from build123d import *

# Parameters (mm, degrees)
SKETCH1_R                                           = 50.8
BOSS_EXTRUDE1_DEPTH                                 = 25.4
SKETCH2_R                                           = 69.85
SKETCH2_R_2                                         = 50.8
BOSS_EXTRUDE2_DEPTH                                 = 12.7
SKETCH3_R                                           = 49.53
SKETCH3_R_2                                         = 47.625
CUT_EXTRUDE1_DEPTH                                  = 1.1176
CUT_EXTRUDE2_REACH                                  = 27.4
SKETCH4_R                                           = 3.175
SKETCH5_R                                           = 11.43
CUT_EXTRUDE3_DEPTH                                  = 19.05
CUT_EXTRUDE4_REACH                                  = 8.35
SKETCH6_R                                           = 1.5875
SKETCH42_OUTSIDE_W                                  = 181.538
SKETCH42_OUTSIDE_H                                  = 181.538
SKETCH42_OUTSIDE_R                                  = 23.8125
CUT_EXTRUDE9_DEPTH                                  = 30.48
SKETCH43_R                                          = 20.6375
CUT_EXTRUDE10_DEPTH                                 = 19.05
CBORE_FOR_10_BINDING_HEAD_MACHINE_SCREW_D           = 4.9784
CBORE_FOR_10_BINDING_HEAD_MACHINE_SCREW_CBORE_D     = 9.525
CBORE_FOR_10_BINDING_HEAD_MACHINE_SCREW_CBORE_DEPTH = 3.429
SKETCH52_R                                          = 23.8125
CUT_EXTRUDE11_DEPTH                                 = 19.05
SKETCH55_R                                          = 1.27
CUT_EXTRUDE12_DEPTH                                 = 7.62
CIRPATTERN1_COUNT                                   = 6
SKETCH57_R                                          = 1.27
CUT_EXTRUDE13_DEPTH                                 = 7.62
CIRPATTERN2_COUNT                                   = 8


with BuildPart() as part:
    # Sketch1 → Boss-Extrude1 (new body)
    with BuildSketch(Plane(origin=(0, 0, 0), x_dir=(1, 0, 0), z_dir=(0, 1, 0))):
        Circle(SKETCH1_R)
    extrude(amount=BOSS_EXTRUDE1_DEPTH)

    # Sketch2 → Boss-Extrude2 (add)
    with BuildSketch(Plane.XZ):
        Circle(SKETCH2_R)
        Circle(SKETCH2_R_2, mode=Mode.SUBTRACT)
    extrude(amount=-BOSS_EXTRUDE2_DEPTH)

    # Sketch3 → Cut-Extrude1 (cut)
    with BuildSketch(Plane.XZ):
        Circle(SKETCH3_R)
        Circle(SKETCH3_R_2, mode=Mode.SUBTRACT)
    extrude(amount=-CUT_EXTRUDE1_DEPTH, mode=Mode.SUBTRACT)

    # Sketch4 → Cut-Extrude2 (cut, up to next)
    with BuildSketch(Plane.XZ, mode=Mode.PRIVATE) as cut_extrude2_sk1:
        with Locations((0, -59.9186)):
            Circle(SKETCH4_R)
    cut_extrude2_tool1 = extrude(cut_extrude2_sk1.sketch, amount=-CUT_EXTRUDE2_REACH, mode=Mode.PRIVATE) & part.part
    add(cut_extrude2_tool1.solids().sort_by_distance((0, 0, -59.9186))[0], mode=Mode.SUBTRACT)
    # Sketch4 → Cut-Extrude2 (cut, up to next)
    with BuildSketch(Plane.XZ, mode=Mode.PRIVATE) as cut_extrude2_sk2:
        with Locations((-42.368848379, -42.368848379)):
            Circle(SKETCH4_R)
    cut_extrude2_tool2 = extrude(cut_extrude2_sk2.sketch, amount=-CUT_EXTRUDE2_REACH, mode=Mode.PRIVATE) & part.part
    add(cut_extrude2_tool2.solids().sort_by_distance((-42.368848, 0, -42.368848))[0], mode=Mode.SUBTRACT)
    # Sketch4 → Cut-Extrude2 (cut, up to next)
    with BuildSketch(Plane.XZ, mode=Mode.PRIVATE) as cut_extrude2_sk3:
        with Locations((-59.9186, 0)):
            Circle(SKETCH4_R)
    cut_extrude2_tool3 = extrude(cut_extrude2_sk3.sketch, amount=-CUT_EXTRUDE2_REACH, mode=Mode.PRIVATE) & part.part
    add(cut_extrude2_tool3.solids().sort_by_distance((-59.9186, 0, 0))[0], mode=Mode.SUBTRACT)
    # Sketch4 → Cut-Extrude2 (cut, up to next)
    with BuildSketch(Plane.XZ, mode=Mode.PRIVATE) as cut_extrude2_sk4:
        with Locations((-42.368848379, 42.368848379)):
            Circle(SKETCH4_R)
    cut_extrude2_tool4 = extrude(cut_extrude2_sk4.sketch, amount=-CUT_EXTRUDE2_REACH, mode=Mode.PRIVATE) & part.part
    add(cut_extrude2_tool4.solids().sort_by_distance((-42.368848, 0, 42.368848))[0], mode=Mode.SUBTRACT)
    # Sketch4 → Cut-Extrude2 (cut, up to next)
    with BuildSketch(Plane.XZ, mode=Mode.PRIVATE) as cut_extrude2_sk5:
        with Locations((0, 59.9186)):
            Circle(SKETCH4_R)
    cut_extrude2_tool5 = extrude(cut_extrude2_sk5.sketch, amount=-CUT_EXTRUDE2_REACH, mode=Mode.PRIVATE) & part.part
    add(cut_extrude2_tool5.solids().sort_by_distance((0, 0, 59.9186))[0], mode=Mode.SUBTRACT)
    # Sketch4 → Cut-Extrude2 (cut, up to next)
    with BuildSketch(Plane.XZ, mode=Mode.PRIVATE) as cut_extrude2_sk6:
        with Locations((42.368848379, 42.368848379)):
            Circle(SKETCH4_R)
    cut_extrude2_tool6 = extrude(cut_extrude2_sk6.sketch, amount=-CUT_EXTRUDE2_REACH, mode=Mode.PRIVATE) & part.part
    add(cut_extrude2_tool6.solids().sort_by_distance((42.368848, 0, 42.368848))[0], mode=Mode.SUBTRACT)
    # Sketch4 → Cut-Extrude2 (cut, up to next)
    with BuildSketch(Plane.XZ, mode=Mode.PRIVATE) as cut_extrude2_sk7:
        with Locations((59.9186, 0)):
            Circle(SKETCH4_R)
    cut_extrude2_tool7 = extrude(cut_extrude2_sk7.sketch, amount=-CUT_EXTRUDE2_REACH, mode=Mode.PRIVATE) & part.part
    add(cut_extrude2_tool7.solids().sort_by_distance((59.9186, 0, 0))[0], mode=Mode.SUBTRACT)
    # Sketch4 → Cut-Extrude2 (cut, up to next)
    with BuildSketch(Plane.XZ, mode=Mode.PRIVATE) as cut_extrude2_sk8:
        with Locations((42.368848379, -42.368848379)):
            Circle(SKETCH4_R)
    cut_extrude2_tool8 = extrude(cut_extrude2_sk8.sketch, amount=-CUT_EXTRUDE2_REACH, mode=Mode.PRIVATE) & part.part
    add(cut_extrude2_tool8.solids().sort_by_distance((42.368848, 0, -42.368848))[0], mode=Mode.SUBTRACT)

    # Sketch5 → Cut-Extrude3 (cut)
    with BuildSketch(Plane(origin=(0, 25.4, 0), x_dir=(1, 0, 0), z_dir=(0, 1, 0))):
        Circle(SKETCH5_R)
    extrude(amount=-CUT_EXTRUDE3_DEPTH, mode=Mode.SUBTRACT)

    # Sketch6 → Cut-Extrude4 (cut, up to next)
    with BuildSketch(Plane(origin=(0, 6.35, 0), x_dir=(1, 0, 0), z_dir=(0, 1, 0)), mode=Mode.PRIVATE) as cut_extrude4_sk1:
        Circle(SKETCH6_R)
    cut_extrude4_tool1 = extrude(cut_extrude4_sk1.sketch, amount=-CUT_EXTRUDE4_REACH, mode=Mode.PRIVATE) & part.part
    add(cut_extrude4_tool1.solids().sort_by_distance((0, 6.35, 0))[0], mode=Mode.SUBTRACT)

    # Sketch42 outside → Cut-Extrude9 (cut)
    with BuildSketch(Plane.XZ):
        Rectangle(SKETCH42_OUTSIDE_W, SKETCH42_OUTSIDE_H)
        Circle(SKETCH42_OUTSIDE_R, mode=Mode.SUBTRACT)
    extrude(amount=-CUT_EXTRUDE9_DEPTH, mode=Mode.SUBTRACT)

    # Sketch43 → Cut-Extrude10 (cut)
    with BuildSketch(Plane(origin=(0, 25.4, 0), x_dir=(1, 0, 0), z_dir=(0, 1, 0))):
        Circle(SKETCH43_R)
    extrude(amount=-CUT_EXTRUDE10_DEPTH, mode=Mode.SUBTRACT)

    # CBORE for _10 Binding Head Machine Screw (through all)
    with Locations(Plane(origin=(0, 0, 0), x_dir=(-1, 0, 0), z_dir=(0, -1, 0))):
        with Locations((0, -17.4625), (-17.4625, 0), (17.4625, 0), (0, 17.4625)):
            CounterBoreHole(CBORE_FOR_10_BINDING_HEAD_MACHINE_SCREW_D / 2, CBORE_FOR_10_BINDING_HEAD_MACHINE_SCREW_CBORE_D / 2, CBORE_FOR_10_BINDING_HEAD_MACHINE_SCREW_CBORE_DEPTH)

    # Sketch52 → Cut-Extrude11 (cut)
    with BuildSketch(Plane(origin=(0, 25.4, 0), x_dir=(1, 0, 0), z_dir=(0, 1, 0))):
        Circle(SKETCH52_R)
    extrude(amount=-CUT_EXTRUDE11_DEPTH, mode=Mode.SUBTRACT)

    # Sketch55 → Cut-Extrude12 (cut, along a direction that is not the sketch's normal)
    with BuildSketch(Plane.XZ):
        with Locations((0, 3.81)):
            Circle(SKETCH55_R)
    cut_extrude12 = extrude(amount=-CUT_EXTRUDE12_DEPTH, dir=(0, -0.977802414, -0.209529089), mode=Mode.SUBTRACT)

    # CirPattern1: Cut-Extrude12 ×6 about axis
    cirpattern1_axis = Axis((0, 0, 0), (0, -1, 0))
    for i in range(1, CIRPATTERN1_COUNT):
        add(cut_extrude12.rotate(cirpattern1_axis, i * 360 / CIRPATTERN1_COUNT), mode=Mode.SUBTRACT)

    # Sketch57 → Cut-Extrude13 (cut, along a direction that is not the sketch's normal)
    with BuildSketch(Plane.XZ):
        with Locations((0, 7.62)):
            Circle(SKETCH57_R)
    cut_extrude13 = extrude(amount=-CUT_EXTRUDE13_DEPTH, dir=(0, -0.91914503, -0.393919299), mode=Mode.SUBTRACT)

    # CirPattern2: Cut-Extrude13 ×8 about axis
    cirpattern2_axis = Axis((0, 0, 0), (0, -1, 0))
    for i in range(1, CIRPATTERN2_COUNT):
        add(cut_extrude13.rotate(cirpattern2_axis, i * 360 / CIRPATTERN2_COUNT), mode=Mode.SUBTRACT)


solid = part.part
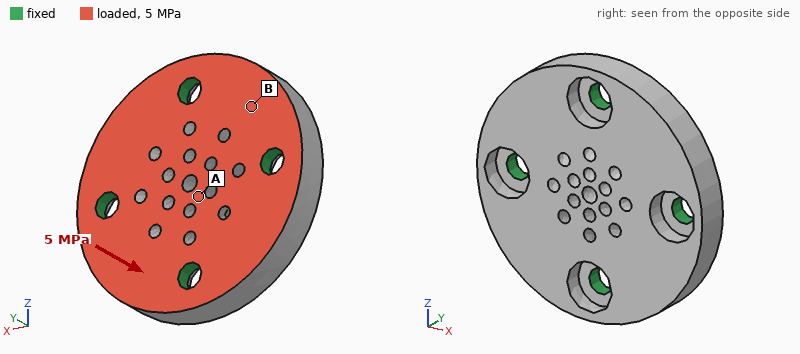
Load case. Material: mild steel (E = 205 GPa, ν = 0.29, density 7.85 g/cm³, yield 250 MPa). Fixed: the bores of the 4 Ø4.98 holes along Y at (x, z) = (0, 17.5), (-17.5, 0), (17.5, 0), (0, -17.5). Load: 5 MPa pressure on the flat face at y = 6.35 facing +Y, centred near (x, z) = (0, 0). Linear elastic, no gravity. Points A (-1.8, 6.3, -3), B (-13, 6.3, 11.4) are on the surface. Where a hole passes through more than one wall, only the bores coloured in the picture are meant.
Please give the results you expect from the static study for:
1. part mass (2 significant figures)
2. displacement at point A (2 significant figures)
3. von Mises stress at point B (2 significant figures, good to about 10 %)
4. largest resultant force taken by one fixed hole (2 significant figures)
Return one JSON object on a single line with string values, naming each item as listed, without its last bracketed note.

{"part mass": "75 g", "displacement at point A": "4.1 µm", "von Mises stress at point B": "23 MPa", "largest resultant force taken by one fixed hole": "2.1 kN"}
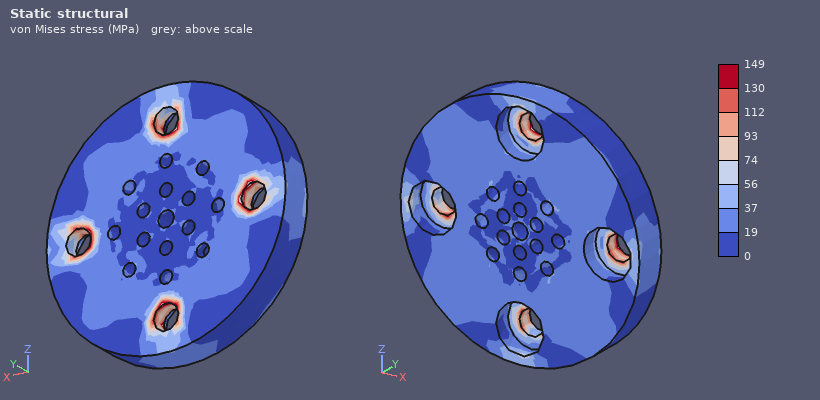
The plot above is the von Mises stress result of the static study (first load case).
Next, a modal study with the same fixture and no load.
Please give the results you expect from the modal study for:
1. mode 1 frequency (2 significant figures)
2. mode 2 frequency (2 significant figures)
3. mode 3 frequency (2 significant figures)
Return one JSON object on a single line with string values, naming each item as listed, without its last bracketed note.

{"mode 1 frequency": "21 kHz", "mode 2 frequency": "23 kHz", "mode 3 frequency": "23 kHz"}
